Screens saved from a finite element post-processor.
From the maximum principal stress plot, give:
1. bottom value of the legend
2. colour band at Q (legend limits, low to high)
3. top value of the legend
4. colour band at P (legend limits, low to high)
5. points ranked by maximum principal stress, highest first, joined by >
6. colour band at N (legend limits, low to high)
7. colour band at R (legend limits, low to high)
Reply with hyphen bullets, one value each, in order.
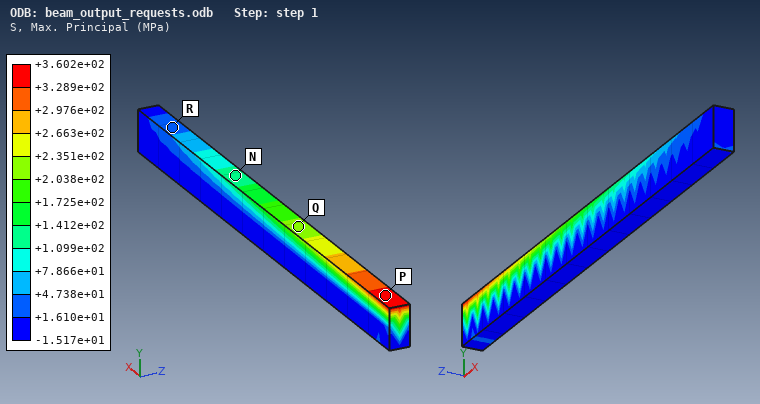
- -1.517e+01 MPa
- +2.038e+02 to +2.351e+02 MPa
- +3.602e+02 MPa
- +3.289e+02 to +3.602e+02 MPa
- P > Q > N > R
- +1.099e+02 to +1.412e+02 MPa
- +1.610e+01 to +4.738e+01 MPa
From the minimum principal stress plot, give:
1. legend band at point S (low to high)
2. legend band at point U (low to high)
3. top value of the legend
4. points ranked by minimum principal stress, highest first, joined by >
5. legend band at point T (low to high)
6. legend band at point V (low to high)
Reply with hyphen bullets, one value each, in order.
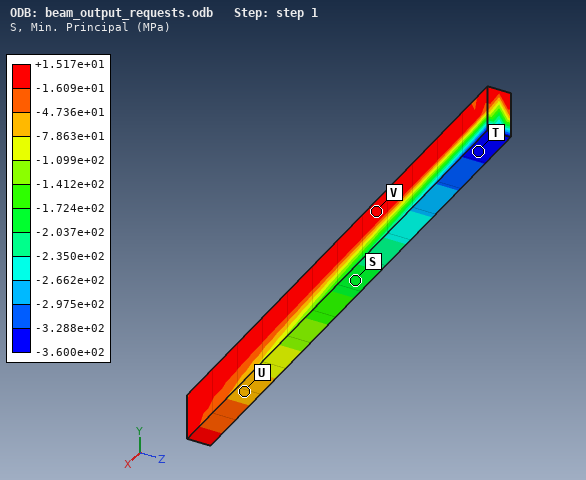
- -2.037e+02 to -1.724e+02 MPa
- -7.863e+01 to -4.736e+01 MPa
- +1.517e+01 MPa
- V > U > S > T
- -3.600e+02 to -3.288e+02 MPa
- -1.609e+01 to +1.517e+01 MPa
